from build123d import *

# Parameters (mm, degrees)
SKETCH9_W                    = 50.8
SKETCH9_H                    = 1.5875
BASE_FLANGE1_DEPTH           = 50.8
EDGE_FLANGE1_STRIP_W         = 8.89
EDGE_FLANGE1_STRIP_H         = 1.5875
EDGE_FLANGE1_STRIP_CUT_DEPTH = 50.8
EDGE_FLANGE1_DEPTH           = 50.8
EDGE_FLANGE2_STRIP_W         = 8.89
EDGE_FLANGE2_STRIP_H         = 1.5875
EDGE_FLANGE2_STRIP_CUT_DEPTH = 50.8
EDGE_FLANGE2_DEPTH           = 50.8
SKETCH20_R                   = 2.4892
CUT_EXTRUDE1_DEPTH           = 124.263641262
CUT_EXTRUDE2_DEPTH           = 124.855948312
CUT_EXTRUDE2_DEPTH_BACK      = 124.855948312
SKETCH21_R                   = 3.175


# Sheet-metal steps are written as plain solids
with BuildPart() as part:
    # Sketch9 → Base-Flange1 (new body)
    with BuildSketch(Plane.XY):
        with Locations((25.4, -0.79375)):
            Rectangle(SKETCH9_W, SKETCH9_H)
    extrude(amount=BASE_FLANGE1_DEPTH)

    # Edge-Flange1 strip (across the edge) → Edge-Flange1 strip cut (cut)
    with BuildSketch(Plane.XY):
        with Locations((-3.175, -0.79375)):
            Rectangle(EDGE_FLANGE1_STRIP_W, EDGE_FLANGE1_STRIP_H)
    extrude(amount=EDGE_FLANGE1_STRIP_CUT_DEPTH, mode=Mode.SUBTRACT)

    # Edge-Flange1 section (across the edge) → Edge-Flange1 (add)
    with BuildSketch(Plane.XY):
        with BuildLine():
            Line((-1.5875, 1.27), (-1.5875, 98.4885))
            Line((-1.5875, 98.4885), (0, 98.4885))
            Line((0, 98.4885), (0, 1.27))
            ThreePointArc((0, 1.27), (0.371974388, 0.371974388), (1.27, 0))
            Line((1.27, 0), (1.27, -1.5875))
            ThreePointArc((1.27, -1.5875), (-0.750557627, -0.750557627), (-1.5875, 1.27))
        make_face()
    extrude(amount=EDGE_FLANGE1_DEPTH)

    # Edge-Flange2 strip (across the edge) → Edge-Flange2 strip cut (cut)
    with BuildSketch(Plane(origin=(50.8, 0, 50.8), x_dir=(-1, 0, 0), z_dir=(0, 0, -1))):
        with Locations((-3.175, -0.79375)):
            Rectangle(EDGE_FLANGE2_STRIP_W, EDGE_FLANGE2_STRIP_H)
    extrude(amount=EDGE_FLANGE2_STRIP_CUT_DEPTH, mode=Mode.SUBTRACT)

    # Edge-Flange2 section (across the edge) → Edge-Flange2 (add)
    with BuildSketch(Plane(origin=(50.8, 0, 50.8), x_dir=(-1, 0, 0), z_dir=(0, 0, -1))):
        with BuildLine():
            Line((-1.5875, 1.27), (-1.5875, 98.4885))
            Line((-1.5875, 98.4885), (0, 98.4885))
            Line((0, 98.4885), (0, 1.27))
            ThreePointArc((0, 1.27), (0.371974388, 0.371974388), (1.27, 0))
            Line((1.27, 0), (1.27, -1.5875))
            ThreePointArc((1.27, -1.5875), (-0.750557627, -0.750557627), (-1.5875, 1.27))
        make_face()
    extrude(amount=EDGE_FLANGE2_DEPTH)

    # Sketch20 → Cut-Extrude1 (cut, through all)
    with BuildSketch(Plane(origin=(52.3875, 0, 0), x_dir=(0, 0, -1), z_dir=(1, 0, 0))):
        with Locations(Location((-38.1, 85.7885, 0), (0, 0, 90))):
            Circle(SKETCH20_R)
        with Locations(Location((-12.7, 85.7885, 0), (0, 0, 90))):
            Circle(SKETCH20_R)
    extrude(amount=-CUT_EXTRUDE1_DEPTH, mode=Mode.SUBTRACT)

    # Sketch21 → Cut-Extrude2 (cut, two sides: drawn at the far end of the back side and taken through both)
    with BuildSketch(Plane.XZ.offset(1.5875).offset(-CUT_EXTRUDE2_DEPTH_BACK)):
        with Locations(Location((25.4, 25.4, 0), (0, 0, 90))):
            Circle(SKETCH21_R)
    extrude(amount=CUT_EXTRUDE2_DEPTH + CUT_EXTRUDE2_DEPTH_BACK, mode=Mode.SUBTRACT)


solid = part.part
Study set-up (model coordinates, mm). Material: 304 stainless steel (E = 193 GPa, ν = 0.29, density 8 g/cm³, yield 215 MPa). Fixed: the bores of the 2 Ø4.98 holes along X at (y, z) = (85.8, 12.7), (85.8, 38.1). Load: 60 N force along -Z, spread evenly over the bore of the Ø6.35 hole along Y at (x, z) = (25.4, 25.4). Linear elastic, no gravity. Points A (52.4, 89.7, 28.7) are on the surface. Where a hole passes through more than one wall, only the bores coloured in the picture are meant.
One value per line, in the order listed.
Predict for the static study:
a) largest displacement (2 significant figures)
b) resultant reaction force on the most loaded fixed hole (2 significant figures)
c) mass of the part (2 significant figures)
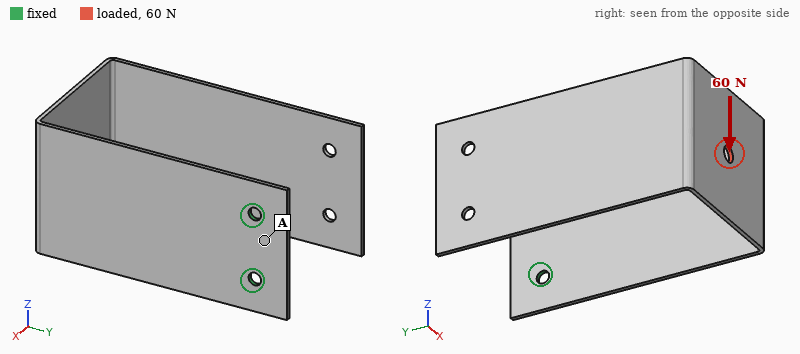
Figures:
1.5 mm
190 N
160 g
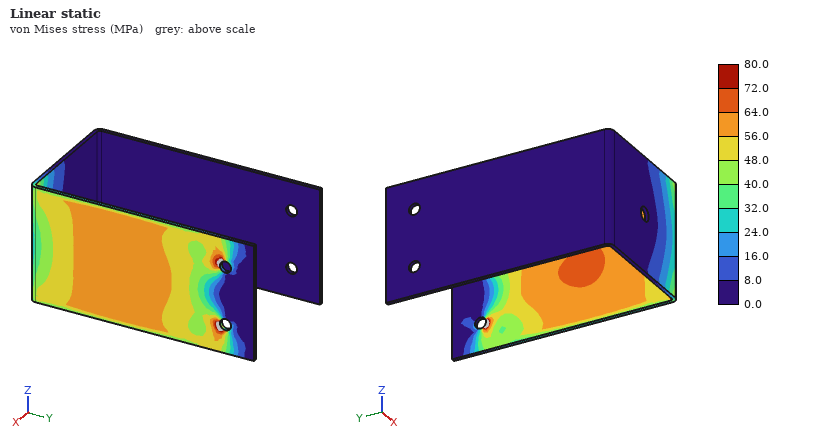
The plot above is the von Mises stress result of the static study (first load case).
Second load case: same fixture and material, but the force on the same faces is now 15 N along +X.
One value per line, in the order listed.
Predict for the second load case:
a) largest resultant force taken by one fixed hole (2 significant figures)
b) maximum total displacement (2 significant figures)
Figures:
7.5 N
1.3 mm
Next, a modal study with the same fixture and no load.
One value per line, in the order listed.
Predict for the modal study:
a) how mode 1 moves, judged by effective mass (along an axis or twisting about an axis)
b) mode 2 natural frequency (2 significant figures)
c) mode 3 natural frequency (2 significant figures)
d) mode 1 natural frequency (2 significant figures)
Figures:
along Y
72 Hz
75 Hz
48 Hz
